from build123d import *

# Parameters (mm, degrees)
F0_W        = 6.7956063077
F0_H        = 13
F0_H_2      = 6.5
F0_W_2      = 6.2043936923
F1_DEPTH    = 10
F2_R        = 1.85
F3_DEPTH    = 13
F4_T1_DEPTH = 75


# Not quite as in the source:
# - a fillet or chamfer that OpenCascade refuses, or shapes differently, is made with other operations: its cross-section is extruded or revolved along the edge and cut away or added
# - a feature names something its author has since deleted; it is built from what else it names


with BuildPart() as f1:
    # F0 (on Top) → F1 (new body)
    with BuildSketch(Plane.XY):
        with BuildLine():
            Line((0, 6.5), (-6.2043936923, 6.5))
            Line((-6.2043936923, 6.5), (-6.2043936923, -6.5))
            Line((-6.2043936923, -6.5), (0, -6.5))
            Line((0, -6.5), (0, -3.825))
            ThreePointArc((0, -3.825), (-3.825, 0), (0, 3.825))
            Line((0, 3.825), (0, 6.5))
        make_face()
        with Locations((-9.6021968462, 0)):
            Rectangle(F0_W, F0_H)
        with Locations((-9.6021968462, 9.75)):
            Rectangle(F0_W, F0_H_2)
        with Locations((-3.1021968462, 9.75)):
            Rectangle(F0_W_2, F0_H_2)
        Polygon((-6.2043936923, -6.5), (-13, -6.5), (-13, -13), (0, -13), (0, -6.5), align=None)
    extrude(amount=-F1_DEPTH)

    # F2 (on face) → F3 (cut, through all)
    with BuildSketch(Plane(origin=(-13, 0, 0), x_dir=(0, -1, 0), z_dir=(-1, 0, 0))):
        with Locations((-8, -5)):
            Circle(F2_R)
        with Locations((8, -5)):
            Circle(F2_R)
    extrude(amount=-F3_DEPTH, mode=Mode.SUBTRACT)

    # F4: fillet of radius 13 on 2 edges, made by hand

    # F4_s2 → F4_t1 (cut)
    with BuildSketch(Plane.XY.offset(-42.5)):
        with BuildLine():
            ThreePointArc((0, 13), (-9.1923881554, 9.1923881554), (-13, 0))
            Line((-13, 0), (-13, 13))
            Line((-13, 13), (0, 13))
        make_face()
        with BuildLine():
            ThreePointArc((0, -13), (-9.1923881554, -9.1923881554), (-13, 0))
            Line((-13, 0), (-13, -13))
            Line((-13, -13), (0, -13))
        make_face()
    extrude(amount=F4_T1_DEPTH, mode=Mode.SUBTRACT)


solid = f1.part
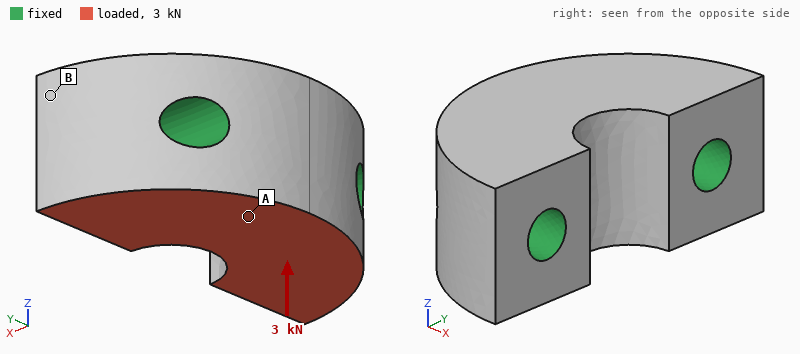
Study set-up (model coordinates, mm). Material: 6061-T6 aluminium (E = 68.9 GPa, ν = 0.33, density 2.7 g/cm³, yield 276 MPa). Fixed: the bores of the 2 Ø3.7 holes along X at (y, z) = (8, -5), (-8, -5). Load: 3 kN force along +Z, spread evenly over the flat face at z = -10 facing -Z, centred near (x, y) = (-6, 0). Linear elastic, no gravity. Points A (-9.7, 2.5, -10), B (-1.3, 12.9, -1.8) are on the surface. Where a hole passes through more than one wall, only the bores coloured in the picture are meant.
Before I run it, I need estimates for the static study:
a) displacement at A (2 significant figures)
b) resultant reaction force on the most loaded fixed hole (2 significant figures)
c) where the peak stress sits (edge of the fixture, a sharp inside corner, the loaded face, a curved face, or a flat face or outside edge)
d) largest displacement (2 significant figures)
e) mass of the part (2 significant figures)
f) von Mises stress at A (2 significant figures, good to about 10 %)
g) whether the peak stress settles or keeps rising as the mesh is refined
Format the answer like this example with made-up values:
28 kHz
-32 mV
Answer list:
2.4 µm
1.5 kN
edge of the fixture
3.4 µm
6.0 g
14 MPa
keeps rising
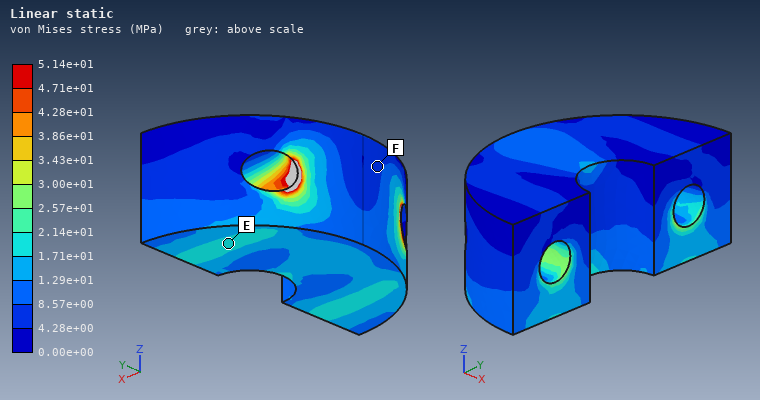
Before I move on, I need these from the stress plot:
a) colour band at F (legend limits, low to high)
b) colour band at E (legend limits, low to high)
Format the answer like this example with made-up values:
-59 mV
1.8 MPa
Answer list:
4.28e+00 to 8.57e+00 MPa
1.71e+01 to 2.14e+01 MPa
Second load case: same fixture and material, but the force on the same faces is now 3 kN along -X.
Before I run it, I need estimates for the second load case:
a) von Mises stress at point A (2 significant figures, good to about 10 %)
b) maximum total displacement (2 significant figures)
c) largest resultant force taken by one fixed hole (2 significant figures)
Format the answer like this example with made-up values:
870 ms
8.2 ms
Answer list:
28 MPa
7.6 µm
1.5 kN
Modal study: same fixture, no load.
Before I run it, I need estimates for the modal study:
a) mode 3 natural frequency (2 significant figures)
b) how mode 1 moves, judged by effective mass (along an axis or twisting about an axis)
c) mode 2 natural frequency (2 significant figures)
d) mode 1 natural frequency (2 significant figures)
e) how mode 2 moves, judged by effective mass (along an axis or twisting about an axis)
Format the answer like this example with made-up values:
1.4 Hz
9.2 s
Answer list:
110 kHz
along Z
95 kHz
79 kHz
along X
